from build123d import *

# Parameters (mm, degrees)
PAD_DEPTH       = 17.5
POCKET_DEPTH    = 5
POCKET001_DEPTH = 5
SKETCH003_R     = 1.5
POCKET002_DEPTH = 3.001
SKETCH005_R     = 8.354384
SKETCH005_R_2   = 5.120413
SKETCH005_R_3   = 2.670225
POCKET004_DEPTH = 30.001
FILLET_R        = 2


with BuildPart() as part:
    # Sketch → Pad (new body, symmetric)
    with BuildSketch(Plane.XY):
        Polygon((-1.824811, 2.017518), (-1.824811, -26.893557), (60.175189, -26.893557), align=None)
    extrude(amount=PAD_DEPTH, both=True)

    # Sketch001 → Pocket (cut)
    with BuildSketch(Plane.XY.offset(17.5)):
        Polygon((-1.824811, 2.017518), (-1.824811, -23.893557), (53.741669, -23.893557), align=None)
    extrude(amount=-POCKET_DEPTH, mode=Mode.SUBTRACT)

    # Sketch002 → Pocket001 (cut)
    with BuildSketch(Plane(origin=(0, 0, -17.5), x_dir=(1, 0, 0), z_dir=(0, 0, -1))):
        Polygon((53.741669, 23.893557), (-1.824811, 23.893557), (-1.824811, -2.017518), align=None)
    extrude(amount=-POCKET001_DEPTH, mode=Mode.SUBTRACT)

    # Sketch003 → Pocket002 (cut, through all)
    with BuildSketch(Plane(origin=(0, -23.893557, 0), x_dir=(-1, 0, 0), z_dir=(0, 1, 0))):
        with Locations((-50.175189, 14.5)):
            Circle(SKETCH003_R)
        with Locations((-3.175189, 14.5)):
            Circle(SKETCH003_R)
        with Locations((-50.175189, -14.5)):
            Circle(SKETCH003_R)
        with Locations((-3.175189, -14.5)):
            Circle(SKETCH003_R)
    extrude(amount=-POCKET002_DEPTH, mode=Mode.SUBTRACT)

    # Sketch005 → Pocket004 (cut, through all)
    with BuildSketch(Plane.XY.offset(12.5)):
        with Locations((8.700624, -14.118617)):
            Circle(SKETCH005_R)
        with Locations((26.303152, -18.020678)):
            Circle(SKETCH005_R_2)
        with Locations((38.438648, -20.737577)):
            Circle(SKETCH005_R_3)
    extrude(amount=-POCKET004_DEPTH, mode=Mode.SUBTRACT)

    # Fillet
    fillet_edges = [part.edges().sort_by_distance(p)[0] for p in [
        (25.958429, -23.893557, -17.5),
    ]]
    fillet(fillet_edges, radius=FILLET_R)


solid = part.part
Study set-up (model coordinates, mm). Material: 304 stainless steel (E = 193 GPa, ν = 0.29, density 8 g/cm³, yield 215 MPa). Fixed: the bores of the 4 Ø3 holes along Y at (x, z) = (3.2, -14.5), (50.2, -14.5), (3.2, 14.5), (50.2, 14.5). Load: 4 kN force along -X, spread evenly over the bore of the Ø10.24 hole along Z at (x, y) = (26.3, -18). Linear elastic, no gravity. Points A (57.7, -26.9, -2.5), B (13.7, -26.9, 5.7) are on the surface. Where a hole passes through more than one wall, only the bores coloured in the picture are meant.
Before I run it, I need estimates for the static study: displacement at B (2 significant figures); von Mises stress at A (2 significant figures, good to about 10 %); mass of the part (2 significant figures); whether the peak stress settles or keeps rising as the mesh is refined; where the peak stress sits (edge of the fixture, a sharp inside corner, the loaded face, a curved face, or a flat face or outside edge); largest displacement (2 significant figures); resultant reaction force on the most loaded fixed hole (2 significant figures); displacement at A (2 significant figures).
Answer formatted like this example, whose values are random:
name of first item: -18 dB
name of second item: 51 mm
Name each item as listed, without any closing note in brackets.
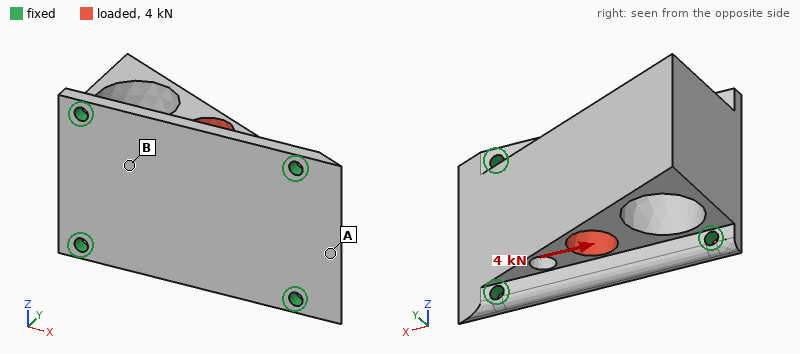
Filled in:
displacement at B: 2.4 µm
von Mises stress at A: 20 MPa
mass of the part: 130 g
whether the peak stress settles or keeps rising as the mesh is refined: keeps rising
where the peak stress sits: edge of the fixture
largest displacement: 5.7 µm
resultant reaction force on the most loaded fixed hole: 1.1 kN
displacement at A: 2.4 µm
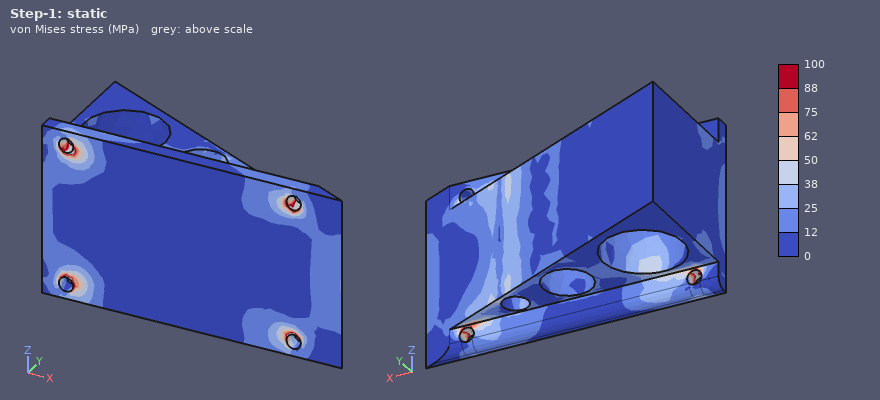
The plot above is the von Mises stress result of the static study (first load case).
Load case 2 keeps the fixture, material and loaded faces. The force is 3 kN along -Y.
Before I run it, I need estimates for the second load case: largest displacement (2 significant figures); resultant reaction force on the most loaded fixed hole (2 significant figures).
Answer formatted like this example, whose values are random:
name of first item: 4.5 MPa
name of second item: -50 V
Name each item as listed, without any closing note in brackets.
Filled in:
largest displacement: 17 µm
resultant reaction force on the most loaded fixed hole: 1.0 kN
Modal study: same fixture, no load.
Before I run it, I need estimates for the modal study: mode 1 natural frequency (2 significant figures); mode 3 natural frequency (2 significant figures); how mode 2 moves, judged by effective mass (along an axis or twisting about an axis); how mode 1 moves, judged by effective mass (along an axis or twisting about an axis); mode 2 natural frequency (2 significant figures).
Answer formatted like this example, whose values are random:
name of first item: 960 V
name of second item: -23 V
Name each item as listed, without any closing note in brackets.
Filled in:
mode 1 natural frequency: 8700 Hz
mode 3 natural frequency: 12 kHz
how mode 2 moves, judged by effective mass: along Z
how mode 1 moves, judged by effective mass: along Y
mode 2 natural frequency: 10 kHz
